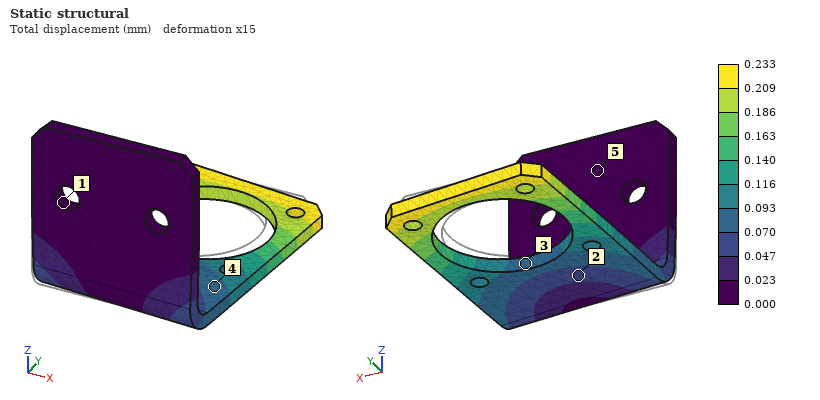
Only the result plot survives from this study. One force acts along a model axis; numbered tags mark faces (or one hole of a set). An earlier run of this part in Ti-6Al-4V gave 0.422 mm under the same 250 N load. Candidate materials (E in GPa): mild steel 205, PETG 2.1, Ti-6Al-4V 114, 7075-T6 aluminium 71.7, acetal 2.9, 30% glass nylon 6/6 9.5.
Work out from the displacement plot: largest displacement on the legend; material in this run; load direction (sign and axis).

0.233 mm
mild steel
+X
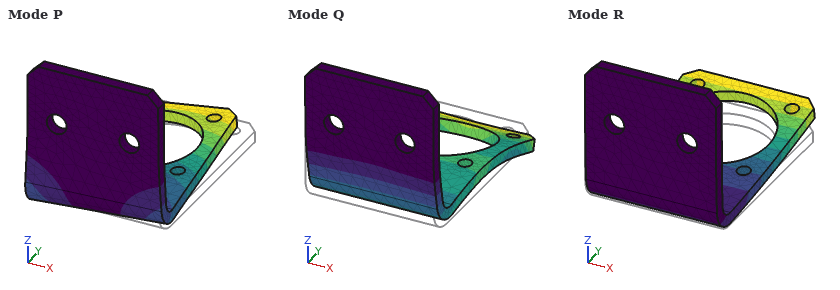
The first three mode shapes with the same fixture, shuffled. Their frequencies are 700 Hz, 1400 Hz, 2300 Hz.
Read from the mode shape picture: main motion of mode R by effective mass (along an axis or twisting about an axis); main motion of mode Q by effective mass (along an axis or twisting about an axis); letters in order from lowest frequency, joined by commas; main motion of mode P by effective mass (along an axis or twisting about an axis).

along Z
along Y
R, P, Q
along X
